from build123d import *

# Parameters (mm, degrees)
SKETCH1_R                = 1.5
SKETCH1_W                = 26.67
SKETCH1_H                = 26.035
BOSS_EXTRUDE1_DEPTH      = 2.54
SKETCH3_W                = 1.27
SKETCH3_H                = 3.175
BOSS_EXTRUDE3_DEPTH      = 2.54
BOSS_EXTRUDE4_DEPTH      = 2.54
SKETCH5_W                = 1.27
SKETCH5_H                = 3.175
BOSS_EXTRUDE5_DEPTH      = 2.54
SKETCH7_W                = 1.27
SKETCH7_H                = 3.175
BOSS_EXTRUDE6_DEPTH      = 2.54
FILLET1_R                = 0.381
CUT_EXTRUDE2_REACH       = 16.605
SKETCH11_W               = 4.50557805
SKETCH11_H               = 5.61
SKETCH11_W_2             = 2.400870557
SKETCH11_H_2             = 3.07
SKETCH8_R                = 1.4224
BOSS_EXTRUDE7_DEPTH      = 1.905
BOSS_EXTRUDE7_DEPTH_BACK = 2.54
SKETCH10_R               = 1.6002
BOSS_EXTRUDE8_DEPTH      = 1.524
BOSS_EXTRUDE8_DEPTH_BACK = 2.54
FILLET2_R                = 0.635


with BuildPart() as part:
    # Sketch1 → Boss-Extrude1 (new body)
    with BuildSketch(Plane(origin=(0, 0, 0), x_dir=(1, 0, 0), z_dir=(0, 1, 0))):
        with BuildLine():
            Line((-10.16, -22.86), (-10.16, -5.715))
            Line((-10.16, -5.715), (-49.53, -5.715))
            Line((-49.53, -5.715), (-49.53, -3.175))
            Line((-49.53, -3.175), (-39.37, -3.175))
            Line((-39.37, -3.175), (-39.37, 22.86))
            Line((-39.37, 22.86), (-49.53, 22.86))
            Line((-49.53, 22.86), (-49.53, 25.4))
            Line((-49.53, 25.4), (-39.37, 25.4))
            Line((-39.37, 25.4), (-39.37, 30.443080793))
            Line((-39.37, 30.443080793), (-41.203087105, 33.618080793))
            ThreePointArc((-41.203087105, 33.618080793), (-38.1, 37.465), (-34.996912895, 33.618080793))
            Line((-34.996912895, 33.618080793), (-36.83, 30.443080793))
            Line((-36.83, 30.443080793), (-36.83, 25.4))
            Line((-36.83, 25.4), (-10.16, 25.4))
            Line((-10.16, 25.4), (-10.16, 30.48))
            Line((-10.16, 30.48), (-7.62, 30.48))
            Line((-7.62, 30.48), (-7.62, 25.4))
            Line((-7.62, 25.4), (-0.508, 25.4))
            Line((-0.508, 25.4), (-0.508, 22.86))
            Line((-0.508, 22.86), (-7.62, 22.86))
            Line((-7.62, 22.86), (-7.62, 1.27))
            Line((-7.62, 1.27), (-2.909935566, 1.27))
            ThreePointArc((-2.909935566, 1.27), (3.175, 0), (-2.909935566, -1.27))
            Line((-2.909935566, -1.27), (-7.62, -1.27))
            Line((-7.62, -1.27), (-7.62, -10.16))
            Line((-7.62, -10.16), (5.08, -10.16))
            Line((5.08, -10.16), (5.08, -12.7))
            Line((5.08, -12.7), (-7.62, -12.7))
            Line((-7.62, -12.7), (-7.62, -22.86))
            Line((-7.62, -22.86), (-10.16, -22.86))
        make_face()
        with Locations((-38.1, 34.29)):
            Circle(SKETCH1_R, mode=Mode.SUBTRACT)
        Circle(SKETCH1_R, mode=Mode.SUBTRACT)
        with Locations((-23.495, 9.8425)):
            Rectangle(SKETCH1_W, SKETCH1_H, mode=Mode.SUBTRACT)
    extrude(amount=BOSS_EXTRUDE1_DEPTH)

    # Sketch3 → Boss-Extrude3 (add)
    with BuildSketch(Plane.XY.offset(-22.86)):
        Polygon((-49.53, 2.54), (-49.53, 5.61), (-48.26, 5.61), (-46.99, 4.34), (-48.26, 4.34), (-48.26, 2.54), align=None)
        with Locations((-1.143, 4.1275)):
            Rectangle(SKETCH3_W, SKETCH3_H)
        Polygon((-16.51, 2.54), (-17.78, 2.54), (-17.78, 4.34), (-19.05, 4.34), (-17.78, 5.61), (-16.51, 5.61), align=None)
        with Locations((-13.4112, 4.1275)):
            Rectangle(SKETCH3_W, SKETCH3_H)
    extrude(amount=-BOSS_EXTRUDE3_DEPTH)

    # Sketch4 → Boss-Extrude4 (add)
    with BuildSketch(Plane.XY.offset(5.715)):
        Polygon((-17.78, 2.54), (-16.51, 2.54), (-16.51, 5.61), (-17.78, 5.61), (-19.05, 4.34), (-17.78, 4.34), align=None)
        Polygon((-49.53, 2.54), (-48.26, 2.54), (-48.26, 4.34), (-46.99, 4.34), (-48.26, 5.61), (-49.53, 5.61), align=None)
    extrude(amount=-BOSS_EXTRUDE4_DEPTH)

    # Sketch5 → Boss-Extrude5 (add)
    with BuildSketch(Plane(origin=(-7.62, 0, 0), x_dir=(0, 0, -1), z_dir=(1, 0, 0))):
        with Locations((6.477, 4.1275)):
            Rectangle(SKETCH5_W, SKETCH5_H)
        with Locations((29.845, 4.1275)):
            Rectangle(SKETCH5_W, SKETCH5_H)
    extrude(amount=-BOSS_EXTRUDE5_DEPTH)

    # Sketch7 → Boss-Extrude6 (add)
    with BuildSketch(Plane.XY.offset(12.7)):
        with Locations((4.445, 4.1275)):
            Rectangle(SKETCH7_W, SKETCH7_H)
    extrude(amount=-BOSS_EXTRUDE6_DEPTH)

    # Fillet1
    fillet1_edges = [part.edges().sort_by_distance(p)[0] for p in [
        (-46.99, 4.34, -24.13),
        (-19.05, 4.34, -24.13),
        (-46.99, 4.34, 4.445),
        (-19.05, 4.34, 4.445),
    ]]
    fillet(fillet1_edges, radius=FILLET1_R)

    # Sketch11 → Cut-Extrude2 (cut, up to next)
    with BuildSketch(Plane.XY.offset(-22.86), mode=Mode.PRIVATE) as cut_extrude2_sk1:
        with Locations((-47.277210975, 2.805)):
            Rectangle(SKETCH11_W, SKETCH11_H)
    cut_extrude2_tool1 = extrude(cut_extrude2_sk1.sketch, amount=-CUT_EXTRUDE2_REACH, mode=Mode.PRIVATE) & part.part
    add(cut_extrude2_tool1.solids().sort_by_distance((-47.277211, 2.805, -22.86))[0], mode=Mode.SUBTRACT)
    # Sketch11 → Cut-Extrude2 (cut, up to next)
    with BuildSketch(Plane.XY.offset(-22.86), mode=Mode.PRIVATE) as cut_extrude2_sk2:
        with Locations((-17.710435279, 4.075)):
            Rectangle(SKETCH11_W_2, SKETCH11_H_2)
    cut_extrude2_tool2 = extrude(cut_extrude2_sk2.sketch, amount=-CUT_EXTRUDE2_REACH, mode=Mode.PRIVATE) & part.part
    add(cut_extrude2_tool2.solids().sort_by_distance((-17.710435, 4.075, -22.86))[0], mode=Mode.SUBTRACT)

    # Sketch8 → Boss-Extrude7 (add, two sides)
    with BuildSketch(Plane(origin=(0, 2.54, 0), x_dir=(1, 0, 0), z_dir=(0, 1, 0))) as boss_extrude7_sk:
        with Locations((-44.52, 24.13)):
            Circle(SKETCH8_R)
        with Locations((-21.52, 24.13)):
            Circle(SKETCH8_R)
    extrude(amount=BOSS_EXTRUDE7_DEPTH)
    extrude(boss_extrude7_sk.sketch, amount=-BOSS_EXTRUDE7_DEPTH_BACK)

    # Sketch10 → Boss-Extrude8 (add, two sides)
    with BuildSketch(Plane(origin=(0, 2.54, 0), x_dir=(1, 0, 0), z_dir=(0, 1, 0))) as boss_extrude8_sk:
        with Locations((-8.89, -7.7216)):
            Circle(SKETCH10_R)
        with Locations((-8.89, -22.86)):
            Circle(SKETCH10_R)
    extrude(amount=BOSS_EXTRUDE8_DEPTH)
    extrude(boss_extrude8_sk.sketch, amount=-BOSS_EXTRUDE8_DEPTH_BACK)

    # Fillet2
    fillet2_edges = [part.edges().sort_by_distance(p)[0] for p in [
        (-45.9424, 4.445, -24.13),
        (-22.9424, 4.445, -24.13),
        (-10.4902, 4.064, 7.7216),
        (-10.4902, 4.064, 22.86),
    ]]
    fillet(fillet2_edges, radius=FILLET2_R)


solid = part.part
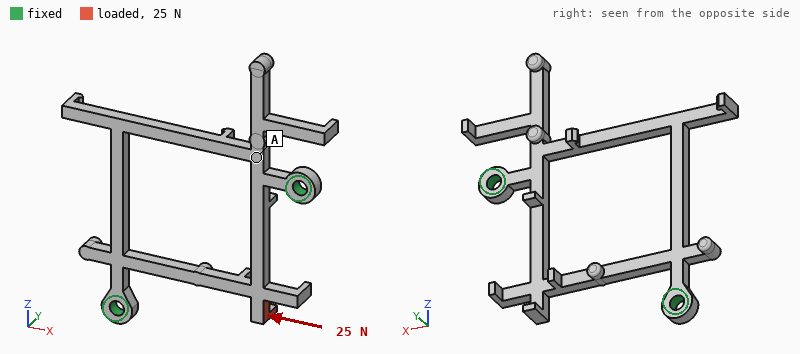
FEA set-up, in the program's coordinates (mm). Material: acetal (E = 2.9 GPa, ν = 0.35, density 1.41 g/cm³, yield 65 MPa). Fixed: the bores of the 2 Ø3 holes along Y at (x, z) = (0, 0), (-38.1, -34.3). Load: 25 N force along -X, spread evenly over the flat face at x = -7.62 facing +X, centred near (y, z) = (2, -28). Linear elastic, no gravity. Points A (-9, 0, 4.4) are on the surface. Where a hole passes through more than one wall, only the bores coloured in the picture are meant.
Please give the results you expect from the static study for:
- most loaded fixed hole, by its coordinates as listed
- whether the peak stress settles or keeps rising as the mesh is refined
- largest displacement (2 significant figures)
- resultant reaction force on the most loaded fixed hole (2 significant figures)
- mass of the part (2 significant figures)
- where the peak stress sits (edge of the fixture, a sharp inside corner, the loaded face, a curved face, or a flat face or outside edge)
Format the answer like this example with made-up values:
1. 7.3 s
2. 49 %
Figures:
1. (-38.1, -34.3)
2. keeps rising
3. 0.91 mm
4. 25 N
5. 2.0 g
6. a sharp inside corner
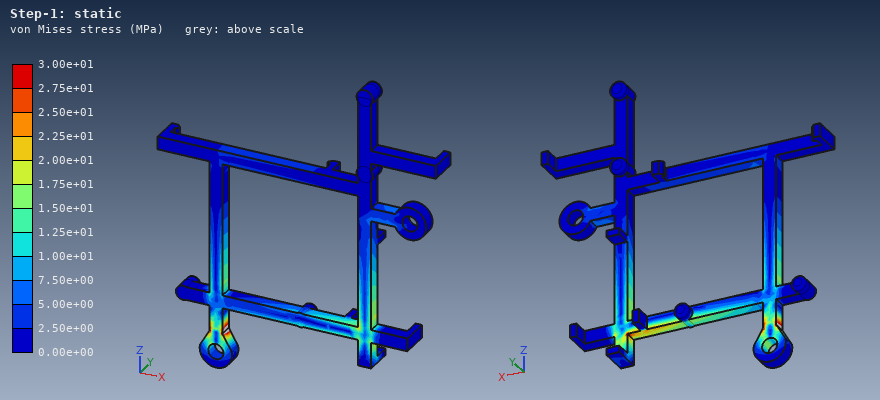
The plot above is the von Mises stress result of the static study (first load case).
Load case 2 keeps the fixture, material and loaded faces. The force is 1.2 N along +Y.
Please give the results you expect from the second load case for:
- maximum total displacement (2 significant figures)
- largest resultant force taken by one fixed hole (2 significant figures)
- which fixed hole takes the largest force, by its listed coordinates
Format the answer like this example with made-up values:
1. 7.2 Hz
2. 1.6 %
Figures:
1. 0.80 mm
2. 0.68 N
3. (0, 0)
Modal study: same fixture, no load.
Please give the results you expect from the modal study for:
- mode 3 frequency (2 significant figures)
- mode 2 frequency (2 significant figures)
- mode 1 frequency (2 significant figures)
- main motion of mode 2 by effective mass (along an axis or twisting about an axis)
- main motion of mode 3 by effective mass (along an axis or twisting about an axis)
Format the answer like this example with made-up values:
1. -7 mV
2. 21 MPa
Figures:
1. 670 Hz
2. 440 Hz
3. 320 Hz
4. along Y
5. along Y
